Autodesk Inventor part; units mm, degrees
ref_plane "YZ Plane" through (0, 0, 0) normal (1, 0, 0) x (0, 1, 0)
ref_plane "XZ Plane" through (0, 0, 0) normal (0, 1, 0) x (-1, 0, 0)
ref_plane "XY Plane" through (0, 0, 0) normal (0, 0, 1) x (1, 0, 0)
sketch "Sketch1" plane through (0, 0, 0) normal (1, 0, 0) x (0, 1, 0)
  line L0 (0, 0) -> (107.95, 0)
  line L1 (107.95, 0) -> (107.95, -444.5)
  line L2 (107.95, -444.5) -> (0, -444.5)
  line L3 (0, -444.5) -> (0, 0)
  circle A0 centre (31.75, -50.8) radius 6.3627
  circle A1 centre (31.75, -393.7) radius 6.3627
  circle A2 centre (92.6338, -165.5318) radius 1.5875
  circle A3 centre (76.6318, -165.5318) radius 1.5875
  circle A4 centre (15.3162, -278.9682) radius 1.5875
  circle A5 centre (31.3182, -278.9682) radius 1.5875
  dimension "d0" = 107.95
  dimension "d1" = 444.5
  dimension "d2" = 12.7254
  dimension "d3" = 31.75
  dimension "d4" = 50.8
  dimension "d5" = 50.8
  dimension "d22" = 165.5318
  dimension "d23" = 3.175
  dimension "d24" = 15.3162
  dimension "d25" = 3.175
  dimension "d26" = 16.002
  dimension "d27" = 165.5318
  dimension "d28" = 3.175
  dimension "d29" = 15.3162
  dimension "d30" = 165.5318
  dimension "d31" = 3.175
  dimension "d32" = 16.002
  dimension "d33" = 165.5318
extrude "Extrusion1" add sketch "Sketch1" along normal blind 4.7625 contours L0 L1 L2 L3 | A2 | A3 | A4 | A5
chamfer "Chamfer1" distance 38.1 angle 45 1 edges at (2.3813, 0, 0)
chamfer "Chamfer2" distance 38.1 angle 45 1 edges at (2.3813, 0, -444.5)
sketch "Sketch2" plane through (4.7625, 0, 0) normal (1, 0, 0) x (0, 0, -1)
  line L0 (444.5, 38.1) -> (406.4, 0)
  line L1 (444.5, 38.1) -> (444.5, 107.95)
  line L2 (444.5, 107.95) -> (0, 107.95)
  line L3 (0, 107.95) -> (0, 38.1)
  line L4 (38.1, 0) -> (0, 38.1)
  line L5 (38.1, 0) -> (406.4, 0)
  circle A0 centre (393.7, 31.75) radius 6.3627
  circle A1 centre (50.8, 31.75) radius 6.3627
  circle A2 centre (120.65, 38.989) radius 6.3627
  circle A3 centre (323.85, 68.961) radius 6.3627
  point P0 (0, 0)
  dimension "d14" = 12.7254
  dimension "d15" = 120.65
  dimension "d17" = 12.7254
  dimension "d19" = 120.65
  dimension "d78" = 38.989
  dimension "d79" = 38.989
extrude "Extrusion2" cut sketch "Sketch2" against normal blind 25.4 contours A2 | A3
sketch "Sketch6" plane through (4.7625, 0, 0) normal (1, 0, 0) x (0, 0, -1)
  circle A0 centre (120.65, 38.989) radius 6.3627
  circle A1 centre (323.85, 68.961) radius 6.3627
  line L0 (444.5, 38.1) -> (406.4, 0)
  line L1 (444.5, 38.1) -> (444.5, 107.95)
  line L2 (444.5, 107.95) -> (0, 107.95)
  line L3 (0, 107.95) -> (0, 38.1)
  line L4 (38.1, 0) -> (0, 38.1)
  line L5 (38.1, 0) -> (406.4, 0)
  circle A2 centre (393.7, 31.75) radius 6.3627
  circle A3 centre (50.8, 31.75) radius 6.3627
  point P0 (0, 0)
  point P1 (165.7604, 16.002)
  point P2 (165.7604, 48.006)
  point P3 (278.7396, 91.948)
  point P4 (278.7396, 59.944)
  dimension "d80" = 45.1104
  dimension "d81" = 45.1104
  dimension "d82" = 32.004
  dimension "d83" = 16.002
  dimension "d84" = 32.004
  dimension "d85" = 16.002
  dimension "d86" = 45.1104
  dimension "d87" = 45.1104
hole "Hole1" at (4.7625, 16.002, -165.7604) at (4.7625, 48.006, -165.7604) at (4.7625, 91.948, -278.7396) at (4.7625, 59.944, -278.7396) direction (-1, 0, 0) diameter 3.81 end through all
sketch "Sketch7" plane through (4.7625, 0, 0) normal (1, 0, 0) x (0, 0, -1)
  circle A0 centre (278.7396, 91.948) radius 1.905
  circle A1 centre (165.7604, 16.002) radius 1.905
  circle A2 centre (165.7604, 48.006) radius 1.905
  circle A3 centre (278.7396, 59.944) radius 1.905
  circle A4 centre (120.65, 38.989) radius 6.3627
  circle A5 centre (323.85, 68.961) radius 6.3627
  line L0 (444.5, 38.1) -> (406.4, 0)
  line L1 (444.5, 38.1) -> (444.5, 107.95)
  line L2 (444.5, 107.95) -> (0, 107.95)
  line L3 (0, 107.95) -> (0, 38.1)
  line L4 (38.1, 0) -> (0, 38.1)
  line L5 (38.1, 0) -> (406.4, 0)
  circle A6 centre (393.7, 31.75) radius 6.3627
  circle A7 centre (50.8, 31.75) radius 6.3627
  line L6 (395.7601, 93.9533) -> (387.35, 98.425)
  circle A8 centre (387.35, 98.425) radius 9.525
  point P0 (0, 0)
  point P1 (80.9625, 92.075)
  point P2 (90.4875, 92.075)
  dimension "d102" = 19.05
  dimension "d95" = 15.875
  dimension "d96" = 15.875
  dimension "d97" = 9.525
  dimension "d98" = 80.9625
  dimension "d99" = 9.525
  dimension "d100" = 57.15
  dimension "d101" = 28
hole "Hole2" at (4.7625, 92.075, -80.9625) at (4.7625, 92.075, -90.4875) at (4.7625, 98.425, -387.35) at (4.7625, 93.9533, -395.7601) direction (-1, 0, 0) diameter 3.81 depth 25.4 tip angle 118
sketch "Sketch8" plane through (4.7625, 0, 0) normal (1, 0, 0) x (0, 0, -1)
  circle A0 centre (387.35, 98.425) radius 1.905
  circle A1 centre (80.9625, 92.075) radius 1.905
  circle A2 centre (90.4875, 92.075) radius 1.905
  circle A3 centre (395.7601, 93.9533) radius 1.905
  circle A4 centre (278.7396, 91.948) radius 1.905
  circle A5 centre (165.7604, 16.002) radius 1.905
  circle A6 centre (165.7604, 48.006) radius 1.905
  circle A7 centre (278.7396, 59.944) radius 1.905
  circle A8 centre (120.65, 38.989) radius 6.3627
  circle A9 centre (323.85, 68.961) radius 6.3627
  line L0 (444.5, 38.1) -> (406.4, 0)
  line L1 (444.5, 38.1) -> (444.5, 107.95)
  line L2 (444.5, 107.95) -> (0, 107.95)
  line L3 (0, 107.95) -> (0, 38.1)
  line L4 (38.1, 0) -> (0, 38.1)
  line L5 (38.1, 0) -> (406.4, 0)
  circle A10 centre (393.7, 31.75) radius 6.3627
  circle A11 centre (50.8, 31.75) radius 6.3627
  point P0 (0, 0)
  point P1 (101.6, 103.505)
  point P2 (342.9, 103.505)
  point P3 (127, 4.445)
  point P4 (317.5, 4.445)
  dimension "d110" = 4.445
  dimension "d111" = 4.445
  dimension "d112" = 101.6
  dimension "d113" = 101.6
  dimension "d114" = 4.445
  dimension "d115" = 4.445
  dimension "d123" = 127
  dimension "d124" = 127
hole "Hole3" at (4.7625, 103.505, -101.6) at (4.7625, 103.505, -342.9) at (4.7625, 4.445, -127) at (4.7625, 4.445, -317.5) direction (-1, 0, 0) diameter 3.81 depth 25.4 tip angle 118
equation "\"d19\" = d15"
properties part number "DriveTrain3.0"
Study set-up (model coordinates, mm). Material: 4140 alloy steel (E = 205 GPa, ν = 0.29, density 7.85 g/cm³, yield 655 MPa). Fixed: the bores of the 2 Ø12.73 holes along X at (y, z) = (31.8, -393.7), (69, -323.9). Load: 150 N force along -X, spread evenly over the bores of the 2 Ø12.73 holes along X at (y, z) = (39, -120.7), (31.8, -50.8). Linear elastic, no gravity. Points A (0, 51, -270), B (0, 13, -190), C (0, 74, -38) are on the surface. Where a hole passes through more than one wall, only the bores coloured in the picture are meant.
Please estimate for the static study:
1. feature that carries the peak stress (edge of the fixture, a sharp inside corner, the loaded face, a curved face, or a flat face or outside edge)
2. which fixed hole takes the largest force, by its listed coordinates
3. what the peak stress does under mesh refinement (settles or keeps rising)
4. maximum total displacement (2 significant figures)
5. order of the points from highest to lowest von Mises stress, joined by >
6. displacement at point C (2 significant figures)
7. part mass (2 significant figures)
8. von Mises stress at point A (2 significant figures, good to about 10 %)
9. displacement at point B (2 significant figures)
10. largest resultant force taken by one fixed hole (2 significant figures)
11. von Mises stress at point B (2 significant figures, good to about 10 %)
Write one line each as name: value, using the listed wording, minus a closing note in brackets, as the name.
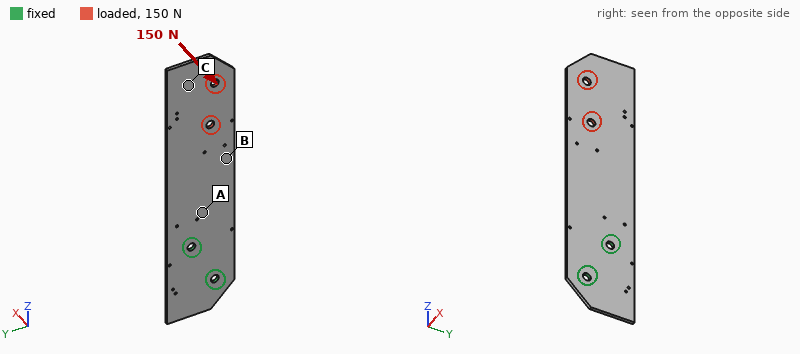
feature that carries the peak stress: edge of the fixture
which fixed hole takes the largest force, by its listed coordinates: (69, -323.9)
what the peak stress does under mesh refinement: keeps rising
maximum total displacement: 5.4 mm
order of the points from highest to lowest von Mises stress, joined by >: A > B > C
displacement at point C: 4.4 mm
part mass: 1.7 kg
von Mises stress at point A: 61 MPa
displacement at point B: 1.4 mm
largest resultant force taken by one fixed hole: 310 N
von Mises stress at point B: 39 MPa
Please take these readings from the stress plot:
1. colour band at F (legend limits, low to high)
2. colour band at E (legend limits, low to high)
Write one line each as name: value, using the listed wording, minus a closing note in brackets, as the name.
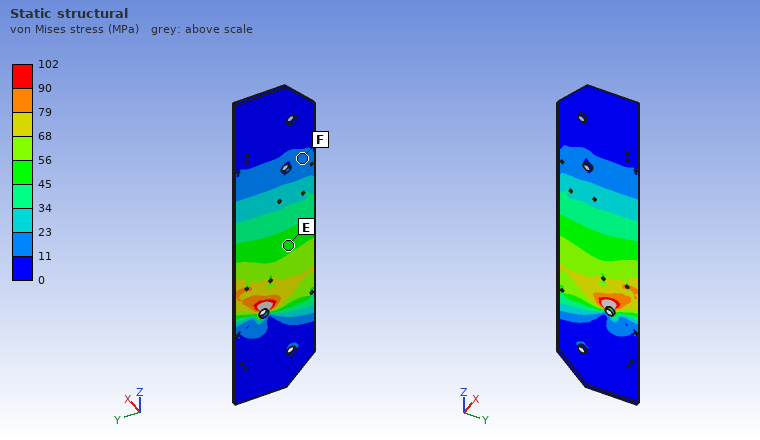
colour band at F: 11 to 23 MPa
colour band at E: 45 to 56 MPa
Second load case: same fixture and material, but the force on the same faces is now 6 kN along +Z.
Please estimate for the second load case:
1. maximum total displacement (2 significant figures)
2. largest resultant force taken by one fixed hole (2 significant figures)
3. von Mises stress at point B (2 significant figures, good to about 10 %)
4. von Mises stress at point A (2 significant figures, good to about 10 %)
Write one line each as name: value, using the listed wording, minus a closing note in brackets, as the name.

maximum total displacement: 85 µm
largest resultant force taken by one fixed hole: 3.3 kN
von Mises stress at point B: 20 MPa
von Mises stress at point A: 14 MPa
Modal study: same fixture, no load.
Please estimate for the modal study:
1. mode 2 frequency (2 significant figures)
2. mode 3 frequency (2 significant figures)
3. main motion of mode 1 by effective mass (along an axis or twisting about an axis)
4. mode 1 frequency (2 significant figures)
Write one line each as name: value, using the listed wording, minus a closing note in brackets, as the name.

mode 2 frequency: 210 Hz
mode 3 frequency: 250 Hz
main motion of mode 1 by effective mass: along X
mode 1 frequency: 39 Hz
